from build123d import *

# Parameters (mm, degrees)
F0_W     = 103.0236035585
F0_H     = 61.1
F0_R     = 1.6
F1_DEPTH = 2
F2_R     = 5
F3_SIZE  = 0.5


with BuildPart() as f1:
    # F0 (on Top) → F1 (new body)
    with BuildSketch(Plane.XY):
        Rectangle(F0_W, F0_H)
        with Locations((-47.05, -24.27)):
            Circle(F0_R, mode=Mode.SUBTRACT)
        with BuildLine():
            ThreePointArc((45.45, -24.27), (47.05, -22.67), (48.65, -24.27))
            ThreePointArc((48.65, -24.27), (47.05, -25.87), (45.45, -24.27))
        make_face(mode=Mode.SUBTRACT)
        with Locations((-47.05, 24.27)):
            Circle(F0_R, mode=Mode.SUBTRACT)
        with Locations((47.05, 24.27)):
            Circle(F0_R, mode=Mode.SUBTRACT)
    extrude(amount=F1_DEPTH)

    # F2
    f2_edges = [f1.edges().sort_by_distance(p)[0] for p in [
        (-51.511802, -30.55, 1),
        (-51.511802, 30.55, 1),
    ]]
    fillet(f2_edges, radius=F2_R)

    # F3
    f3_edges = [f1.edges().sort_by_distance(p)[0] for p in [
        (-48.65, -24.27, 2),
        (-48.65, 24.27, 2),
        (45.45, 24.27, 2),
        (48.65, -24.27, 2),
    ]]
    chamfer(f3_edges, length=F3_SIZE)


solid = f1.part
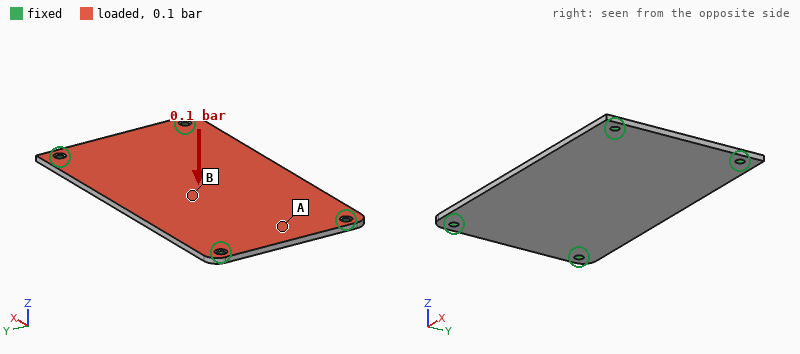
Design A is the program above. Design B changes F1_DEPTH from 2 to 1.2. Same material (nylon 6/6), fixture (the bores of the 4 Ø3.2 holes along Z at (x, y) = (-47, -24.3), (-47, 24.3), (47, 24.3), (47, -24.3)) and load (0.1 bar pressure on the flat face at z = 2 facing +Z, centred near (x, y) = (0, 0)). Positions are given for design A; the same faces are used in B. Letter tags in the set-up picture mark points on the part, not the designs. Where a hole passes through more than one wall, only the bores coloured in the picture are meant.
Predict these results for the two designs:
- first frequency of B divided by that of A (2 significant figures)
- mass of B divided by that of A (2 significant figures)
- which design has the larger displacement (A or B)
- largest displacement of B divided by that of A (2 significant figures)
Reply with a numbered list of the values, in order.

1. 0.60
2. 0.60
3. B
4. 4.6
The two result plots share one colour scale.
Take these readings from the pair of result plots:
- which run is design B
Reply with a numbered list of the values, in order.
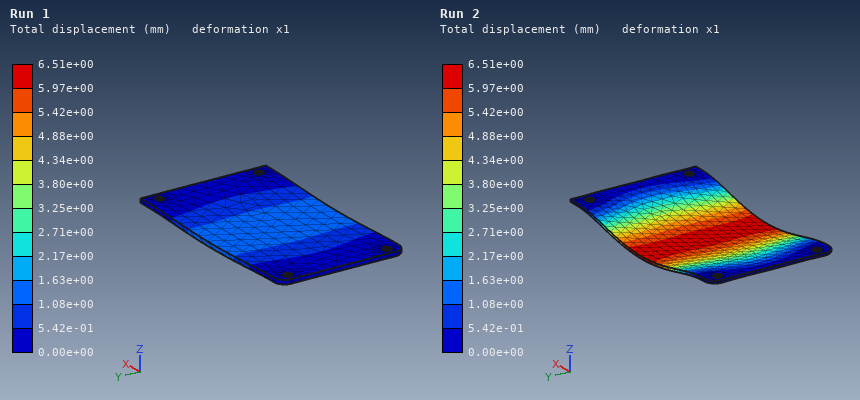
1. Run 2
